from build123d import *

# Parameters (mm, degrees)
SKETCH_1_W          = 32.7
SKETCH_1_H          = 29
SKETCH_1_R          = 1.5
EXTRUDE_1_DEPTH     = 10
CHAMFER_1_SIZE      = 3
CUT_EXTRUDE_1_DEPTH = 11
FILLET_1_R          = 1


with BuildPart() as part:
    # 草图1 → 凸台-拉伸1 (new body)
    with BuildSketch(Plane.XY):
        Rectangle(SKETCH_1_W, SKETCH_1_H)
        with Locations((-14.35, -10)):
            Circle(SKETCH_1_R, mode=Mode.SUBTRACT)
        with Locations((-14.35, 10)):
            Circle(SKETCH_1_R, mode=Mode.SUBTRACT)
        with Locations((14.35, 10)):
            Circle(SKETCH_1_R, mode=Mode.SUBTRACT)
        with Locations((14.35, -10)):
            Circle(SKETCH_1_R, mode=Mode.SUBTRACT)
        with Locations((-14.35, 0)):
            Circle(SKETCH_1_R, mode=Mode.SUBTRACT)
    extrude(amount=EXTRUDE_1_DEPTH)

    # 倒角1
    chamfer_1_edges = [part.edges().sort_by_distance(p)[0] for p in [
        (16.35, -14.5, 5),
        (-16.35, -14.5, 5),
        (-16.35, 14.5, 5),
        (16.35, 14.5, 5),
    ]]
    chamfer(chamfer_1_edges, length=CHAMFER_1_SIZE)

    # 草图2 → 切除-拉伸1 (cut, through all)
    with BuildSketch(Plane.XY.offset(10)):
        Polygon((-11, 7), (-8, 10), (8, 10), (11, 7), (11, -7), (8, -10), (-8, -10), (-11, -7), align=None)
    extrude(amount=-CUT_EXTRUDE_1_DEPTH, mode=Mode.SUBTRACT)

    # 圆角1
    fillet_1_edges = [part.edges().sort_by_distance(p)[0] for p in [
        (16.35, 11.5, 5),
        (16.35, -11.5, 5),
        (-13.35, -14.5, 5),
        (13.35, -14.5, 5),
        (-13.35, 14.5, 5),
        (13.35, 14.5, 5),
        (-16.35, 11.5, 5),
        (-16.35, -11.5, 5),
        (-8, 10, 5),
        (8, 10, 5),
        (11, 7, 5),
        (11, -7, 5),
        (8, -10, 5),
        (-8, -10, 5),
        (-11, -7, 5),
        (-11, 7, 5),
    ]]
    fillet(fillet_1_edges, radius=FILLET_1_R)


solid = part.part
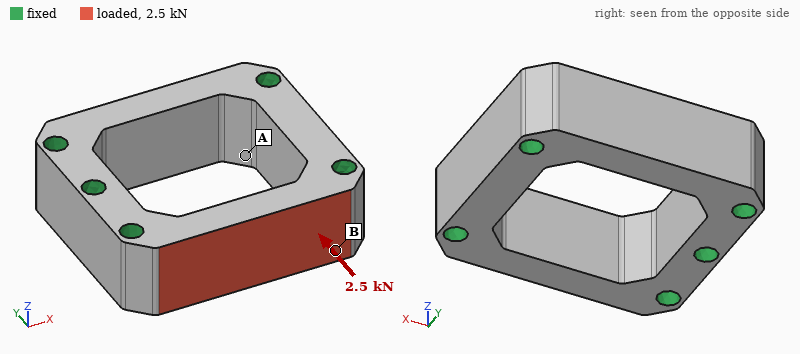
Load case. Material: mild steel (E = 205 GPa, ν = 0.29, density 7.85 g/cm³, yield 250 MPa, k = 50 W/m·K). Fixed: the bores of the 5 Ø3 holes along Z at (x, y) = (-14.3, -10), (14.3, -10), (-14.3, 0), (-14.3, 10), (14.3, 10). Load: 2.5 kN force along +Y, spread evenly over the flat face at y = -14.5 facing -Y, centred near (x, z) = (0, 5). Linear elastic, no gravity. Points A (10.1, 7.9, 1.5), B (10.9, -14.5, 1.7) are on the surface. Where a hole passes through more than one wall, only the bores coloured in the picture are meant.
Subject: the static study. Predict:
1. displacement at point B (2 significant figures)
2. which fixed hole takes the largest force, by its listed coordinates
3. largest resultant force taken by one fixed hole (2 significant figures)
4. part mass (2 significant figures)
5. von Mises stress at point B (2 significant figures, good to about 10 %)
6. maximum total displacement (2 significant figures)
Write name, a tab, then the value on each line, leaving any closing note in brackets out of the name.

displacement at point B	2.0 µm
which fixed hole takes the largest force, by its listed coordinates	(14.3, -10)
largest resultant force taken by one fixed hole	1.2 kN
part mass	37 g
von Mises stress at point B	30 MPa
maximum total displacement	7.1 µm
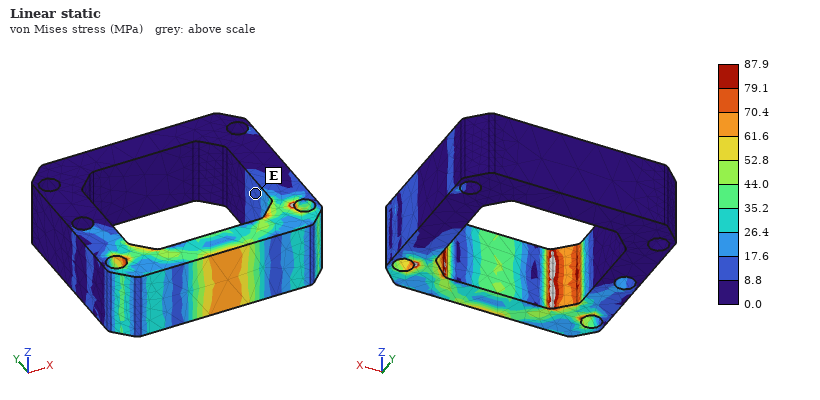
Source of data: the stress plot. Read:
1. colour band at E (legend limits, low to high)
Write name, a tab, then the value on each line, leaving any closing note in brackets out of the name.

colour band at E	8.8 to 17.6 MPa
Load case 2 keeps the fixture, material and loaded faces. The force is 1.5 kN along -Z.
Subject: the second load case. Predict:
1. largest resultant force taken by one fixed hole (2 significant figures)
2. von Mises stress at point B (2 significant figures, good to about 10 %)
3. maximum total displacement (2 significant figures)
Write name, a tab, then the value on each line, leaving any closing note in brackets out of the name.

largest resultant force taken by one fixed hole	770 N
von Mises stress at point B	31 MPa
maximum total displacement	4.3 µm
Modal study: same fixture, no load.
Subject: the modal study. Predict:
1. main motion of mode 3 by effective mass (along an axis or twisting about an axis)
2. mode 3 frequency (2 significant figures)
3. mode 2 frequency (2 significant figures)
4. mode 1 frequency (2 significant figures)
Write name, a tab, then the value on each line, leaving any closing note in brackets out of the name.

main motion of mode 3 by effective mass	along Z
mode 3 frequency	45 kHz
mode 2 frequency	36 kHz
mode 1 frequency	35 kHz
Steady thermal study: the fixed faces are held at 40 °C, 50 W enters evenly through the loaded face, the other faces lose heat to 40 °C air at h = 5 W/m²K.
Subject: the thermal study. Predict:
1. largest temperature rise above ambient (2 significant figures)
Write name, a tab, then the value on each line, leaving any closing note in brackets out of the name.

largest temperature rise above ambient	75 K
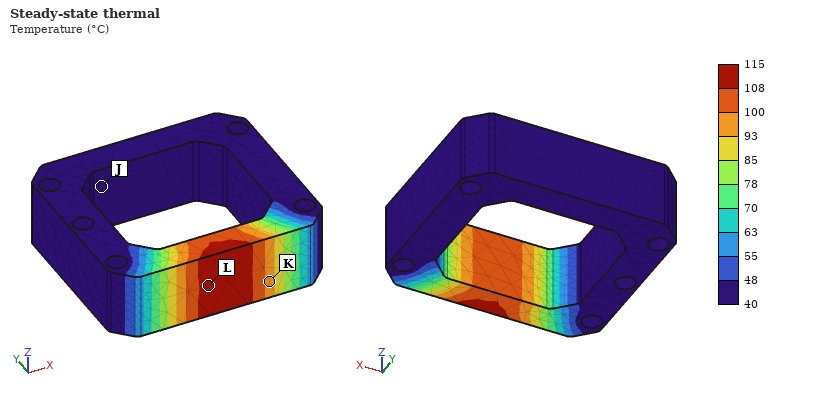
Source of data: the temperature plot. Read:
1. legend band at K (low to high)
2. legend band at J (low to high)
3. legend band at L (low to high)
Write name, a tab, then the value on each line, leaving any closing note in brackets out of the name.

legend band at K	93 to 100 °C
legend band at J	40 to 48 °C
legend band at L	108 to 115 °C
